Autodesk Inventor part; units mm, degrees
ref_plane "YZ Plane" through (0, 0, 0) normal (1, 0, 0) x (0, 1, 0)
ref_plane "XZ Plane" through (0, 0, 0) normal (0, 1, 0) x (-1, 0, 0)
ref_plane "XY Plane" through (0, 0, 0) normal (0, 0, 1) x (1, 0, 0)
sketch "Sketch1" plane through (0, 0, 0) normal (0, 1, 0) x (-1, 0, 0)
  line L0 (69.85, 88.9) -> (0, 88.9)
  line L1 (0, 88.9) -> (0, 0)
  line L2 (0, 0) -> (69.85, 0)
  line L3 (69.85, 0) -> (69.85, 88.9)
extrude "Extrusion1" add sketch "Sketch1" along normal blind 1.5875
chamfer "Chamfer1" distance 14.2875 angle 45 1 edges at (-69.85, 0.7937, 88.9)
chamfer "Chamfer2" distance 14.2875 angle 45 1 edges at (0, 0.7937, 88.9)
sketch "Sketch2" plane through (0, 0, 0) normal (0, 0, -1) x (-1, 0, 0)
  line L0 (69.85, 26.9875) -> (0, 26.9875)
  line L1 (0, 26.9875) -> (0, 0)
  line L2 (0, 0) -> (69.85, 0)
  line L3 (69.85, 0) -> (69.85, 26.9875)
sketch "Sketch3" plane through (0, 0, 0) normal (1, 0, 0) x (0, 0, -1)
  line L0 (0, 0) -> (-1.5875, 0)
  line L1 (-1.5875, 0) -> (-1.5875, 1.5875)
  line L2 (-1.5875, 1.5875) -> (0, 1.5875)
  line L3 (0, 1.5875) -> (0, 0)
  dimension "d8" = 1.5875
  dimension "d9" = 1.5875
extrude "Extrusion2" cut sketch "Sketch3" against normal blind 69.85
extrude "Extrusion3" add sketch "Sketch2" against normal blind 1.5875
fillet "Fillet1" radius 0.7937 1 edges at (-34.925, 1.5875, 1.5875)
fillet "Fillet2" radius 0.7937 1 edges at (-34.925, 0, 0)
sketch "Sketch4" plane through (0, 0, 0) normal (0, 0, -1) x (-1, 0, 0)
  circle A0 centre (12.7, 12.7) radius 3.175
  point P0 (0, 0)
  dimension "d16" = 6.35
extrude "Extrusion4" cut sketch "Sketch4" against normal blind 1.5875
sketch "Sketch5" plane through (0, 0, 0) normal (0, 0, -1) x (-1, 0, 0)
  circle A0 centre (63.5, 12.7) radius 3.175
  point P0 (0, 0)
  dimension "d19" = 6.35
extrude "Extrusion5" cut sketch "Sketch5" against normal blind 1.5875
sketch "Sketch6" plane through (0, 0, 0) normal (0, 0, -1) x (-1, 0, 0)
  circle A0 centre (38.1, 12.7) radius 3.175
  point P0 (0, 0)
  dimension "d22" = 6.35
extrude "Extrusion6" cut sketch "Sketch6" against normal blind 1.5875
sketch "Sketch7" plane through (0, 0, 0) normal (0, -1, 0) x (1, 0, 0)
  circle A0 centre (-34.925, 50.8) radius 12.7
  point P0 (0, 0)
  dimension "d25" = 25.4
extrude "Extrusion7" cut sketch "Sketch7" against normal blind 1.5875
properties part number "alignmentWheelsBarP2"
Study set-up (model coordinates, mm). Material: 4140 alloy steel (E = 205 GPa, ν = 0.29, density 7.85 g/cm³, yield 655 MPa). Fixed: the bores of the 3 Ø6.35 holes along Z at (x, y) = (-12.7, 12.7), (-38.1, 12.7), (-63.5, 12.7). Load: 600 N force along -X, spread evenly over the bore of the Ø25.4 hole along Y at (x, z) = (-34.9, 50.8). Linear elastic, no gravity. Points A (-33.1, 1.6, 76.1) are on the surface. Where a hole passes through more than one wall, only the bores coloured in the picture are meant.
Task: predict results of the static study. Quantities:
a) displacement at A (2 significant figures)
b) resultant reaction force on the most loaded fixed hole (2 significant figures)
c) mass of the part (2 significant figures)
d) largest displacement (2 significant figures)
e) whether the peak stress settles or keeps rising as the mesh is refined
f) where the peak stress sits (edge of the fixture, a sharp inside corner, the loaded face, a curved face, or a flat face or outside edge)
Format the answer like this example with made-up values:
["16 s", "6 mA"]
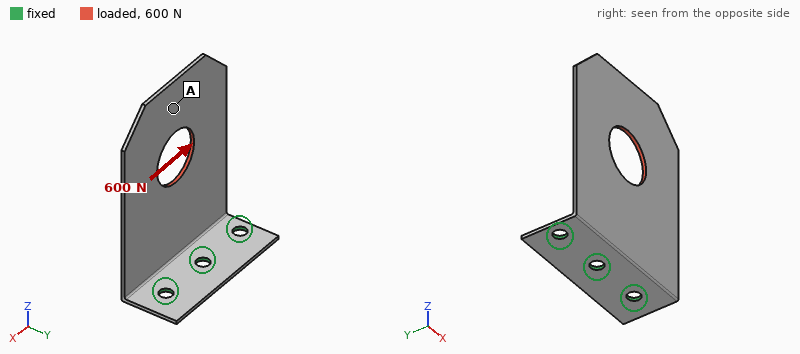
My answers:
["0.29 mm", "620 N", "89 g", "0.43 mm", "keeps rising", "edge of the fixture"]
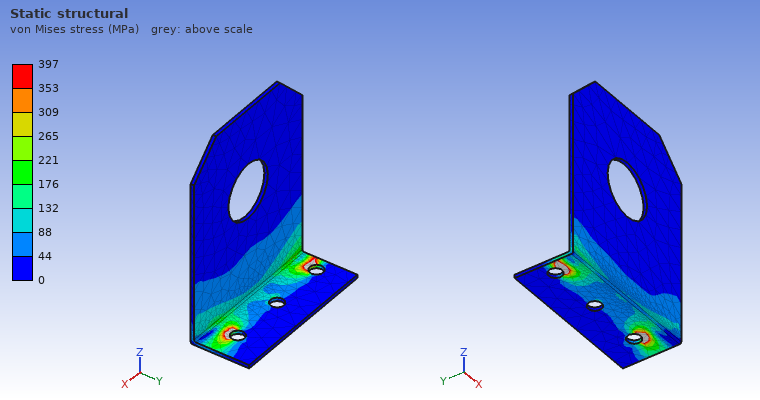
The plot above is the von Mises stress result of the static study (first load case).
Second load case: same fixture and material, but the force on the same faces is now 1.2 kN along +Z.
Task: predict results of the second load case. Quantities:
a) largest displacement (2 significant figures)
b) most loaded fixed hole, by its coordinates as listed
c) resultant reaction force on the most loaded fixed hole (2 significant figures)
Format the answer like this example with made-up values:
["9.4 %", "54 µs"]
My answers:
["1.1 mm", "(-12.7, 12.7)", "460 N"]
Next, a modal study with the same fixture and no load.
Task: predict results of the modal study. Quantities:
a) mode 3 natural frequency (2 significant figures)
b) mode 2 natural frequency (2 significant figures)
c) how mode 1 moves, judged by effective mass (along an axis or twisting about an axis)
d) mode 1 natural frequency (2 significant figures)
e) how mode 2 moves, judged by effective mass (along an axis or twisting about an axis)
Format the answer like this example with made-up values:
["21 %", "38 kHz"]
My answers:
["900 Hz", "490 Hz", "along Y", "160 Hz", "twisting about Z"]
